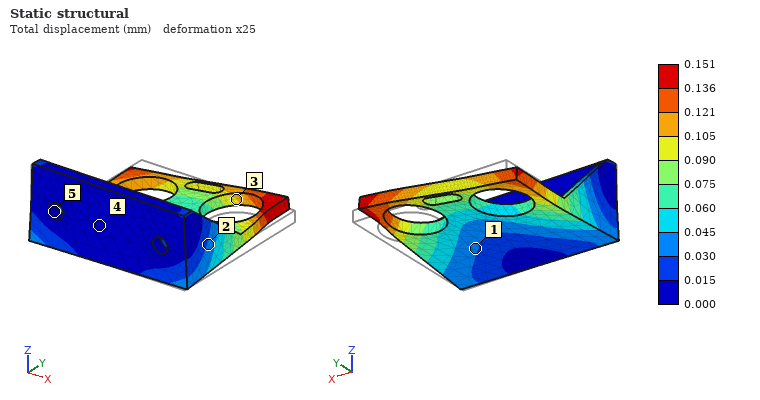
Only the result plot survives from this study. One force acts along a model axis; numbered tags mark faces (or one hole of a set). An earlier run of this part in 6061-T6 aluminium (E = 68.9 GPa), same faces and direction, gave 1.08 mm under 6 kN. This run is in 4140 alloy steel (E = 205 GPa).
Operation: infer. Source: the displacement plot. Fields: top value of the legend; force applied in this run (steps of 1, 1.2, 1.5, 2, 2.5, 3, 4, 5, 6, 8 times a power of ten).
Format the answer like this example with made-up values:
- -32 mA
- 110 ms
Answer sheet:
- 0.151 mm
- 2.5 kN
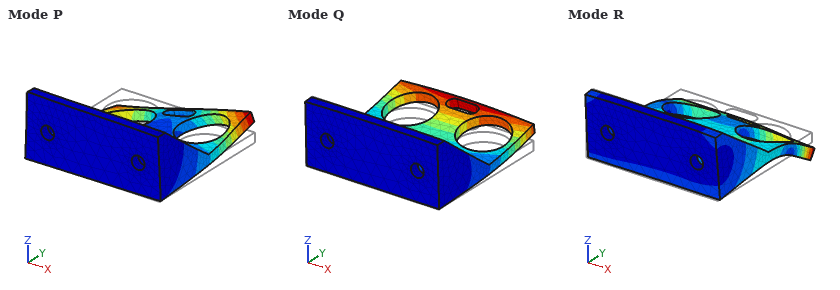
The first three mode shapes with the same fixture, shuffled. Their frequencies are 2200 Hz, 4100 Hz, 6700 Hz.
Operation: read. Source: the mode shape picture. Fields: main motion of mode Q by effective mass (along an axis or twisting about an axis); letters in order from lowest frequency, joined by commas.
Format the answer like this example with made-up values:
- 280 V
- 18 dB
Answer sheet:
- along Z
- Q, P, R
